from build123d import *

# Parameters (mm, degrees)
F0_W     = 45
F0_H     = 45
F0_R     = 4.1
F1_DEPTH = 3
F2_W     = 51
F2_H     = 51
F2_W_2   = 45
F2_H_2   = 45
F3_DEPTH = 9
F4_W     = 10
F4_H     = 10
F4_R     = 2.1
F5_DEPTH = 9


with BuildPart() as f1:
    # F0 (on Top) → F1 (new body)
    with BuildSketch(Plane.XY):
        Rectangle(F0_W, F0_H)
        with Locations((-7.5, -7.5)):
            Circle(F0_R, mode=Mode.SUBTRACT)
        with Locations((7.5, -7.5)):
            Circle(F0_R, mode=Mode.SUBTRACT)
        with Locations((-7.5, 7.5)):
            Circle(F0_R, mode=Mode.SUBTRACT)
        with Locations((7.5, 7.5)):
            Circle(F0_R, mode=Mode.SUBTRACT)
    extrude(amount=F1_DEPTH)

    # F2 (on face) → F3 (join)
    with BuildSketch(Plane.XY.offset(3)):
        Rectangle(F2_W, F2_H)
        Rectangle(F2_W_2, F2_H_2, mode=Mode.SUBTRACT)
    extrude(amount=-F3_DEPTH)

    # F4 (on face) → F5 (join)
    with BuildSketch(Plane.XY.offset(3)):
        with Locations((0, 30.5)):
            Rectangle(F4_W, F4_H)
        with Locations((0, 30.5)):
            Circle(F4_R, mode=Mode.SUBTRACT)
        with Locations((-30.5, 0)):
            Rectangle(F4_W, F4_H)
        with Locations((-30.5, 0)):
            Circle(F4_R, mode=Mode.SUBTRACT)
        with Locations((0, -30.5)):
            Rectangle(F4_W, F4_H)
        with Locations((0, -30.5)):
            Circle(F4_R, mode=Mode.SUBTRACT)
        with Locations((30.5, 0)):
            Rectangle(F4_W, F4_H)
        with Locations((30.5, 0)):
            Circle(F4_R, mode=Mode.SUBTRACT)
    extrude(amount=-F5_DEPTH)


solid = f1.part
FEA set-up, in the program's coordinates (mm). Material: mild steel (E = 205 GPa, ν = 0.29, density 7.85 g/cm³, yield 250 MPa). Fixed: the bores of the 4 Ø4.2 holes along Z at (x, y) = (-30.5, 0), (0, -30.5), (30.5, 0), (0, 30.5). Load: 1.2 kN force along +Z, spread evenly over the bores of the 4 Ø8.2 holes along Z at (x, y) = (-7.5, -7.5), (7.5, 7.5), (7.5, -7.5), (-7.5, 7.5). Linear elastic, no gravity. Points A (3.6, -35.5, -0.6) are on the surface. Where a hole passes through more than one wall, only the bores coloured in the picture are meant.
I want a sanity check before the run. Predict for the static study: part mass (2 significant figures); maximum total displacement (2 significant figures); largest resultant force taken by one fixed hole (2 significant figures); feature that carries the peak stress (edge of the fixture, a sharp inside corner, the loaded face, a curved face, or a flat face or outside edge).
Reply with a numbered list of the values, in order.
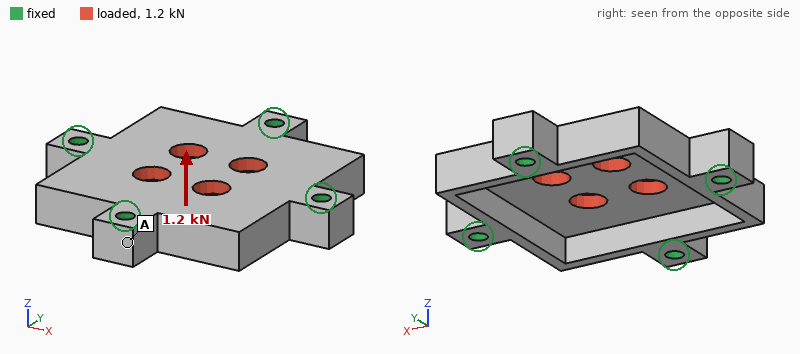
1. 110 g
2. 25 µm
3. 400 N
4. the loaded face
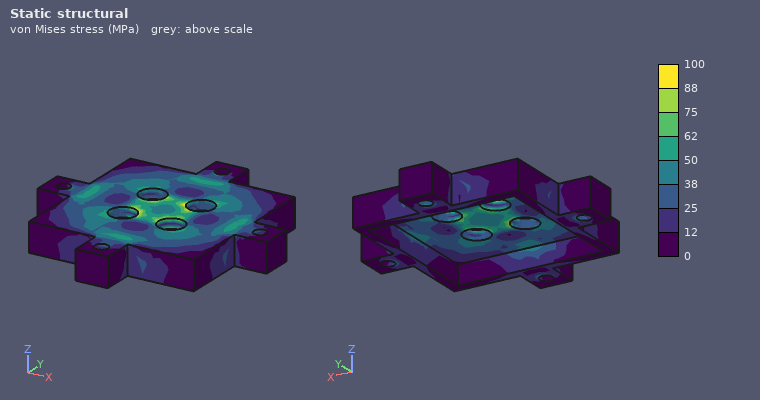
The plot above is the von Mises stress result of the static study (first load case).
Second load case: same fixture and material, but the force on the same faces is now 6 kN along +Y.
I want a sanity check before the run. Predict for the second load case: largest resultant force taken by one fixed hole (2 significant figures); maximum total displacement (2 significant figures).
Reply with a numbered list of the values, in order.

1. 2.0 kN
2. 6.4 µm
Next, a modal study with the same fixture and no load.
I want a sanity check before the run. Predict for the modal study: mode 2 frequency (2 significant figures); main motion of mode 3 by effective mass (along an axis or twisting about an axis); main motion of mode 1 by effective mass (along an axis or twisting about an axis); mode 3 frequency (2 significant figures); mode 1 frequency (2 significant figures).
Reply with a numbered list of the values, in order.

1. 12 kHz
2. twisting about Y
3. along Z
4. 13 kHz
5. 10 kHz
